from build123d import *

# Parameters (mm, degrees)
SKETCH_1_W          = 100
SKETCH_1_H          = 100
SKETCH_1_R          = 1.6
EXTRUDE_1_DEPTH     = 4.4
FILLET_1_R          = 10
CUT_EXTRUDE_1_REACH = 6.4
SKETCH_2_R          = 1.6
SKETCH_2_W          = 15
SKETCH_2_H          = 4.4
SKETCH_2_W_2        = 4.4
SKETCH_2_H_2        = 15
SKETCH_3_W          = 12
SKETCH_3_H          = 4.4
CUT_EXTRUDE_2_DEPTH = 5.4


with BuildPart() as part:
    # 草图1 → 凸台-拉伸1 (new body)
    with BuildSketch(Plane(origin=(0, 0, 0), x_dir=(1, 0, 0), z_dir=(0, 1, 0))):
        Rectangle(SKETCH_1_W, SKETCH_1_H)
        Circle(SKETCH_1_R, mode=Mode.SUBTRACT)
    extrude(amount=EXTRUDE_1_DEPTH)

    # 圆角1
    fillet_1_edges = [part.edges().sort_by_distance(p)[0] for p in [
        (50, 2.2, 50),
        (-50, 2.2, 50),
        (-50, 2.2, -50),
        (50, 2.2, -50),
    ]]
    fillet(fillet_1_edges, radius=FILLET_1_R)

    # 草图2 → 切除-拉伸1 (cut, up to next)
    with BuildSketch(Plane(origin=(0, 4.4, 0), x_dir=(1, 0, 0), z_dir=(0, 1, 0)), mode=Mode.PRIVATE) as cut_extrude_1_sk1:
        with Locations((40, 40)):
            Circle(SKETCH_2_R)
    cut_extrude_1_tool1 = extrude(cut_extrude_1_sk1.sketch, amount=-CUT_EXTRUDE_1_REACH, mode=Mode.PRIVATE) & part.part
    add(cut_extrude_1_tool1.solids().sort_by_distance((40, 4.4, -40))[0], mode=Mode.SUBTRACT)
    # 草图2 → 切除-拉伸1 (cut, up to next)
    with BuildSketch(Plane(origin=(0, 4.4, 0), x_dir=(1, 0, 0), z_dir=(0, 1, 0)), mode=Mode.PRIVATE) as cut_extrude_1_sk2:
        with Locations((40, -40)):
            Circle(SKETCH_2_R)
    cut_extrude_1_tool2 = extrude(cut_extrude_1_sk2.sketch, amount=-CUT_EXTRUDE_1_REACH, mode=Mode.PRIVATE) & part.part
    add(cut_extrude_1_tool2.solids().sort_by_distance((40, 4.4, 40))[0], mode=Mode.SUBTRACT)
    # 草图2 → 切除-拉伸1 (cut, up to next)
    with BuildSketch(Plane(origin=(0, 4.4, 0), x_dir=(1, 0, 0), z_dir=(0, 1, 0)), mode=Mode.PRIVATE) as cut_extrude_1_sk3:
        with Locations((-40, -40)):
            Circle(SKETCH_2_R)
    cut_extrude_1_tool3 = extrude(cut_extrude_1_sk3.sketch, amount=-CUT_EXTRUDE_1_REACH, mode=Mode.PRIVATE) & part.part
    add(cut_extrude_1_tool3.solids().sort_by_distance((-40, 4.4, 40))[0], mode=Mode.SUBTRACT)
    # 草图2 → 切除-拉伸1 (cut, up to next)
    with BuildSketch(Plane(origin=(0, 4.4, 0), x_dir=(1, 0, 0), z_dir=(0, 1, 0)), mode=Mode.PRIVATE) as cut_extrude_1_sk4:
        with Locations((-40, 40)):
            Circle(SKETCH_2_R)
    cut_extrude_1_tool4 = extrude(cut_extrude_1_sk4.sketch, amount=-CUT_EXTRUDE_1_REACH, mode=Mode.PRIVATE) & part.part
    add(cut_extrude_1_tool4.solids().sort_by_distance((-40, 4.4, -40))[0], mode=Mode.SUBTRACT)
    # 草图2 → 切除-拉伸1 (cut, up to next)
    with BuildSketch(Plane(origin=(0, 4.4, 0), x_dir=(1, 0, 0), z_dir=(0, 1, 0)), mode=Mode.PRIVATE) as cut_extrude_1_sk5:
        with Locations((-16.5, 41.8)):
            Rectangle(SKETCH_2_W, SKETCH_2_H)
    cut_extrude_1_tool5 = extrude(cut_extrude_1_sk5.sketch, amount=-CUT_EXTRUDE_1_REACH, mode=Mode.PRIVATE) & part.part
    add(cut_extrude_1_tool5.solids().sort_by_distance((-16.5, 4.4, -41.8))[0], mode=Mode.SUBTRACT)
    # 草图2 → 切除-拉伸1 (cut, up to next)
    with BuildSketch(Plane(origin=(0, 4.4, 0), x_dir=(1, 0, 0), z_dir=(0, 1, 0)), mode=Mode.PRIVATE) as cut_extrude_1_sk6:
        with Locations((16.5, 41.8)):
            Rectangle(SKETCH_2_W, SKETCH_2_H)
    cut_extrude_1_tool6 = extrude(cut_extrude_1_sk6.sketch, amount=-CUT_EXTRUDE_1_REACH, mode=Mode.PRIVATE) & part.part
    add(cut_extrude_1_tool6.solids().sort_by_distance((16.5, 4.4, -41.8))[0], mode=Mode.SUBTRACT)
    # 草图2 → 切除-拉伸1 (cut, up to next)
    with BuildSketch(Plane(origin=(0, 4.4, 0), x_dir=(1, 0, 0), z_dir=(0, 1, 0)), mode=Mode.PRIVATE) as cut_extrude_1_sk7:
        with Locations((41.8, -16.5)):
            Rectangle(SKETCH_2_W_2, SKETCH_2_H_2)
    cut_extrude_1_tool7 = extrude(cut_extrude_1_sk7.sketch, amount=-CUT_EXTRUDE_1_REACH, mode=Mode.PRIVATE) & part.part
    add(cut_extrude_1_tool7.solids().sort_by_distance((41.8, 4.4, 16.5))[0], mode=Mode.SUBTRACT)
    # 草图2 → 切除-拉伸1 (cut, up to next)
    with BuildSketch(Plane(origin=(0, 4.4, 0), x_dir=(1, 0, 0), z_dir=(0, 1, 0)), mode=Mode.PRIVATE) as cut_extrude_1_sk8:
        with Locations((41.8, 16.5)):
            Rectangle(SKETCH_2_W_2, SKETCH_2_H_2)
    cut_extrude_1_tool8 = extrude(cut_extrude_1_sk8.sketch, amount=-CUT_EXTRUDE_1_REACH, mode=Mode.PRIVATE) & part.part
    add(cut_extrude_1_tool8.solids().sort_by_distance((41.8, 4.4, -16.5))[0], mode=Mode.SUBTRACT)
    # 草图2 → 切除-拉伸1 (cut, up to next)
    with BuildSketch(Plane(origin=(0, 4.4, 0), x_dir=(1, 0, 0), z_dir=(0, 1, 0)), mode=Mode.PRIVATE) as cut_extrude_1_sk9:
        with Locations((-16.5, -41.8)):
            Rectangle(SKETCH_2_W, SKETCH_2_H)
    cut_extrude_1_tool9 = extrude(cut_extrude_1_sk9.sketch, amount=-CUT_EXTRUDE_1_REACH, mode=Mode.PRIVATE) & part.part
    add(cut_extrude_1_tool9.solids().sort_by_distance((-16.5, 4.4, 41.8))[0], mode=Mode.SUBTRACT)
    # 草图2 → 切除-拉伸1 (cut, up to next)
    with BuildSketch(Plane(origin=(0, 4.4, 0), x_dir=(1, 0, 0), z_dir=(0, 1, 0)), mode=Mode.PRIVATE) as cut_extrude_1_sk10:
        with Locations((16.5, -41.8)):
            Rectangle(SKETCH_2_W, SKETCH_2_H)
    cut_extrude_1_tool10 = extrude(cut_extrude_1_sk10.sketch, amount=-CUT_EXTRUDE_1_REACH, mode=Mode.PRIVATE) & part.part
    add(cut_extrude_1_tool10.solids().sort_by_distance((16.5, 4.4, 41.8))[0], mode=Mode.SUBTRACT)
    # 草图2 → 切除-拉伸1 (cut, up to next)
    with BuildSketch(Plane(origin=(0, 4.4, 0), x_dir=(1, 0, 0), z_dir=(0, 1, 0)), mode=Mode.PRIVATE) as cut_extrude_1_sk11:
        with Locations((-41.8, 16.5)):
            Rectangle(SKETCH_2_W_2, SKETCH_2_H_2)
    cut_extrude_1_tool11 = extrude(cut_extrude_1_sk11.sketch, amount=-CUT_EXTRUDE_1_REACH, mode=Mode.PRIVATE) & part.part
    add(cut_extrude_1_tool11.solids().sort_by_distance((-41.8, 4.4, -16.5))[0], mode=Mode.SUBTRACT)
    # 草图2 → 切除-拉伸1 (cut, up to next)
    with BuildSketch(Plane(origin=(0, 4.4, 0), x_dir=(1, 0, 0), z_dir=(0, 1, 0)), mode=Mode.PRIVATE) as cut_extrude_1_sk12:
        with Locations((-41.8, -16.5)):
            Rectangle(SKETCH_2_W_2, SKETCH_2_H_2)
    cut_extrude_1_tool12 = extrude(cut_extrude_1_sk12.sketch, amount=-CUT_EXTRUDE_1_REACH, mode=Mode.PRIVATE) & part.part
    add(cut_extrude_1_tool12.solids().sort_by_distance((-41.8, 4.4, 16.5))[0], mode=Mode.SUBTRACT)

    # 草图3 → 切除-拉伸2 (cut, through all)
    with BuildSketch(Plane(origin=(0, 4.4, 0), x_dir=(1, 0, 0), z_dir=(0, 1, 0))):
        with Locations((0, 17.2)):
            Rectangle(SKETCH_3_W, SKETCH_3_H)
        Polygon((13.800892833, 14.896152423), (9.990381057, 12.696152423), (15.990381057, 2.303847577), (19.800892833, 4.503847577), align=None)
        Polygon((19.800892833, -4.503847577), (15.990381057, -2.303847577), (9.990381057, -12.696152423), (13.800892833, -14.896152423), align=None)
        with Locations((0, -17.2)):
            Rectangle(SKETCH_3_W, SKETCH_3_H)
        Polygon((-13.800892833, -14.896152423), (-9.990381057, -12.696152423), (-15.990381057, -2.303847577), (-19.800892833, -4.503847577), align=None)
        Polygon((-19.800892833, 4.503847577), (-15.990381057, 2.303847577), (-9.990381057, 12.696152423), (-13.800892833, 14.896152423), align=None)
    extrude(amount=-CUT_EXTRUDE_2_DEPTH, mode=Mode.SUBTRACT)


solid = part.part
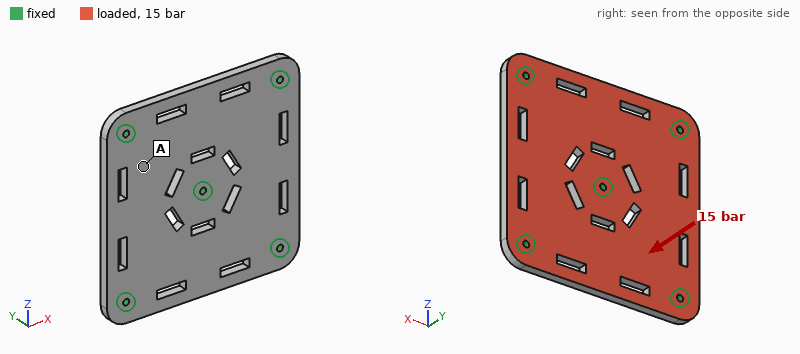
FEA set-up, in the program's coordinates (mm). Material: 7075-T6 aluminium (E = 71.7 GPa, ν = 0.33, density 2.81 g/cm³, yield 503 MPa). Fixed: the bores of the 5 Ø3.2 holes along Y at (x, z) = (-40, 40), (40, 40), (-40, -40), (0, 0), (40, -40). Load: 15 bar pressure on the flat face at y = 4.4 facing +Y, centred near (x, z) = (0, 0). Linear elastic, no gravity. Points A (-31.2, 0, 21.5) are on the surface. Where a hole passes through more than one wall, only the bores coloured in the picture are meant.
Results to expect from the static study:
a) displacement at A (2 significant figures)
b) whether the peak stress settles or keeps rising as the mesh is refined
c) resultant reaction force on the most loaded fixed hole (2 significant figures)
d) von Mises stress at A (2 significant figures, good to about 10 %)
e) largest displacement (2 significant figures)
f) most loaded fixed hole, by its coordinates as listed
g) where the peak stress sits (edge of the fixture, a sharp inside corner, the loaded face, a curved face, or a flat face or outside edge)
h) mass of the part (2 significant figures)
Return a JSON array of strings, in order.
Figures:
["0.14 mm", "keeps rising", "4.5 kN", "86 MPa", "0.26 mm", "(0, 0)", "edge of the fixture", "110 g"]
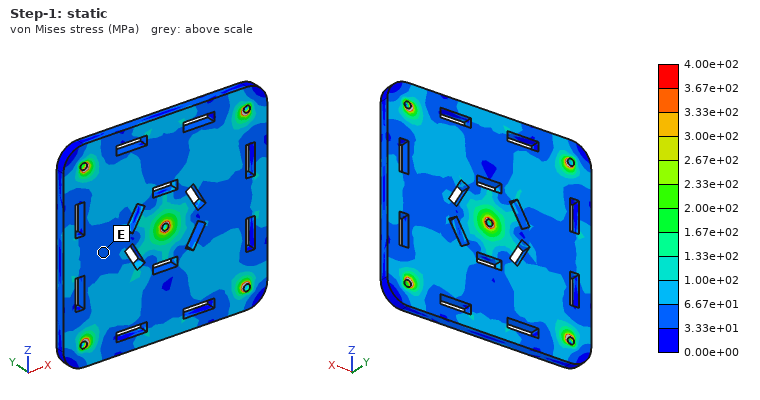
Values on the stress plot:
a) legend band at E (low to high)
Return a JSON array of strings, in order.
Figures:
["3.33e+01 to 6.67e+01 MPa"]
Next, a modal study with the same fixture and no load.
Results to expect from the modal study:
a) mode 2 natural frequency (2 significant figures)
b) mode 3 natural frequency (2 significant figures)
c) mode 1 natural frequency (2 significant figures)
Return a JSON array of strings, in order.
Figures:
["3900 Hz", "3900 Hz", "3800 Hz"]
